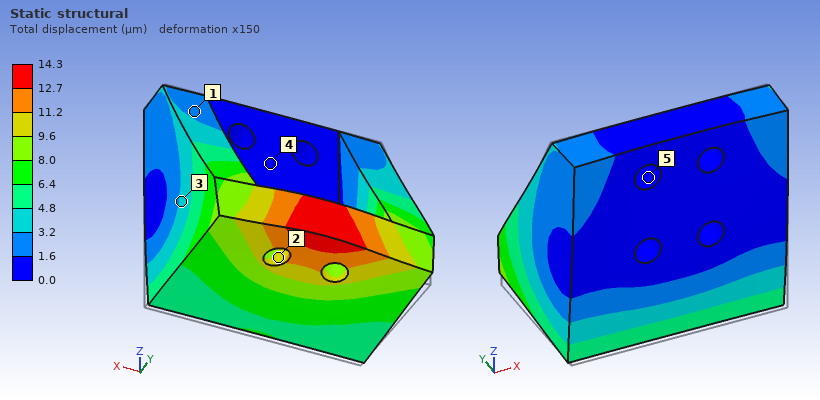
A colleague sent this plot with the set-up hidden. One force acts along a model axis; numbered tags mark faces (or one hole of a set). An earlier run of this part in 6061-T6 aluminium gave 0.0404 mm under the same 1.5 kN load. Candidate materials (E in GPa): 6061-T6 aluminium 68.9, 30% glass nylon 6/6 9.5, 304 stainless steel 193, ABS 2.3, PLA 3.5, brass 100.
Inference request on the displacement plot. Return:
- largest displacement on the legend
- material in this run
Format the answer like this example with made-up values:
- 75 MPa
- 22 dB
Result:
- 14.3 µm
- 304 stainless steel
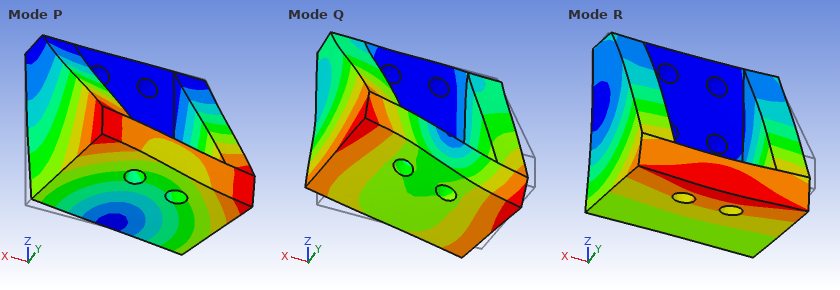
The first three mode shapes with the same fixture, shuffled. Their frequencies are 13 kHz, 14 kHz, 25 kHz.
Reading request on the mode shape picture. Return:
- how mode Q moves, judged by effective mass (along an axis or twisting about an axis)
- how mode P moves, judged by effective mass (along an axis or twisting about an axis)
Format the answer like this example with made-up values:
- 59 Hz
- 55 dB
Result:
- along X
- along X
